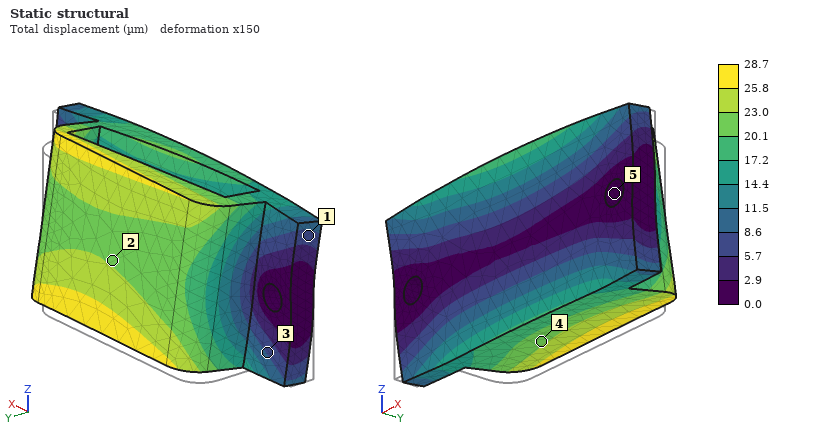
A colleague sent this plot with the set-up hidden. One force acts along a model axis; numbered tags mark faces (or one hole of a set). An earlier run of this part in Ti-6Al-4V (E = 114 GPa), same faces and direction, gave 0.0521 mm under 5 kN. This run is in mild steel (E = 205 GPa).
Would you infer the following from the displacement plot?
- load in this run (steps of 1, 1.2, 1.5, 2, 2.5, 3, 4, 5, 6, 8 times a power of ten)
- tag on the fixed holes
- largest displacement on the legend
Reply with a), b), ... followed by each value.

a) 5 kN
b) 5
c) 28.7 µm
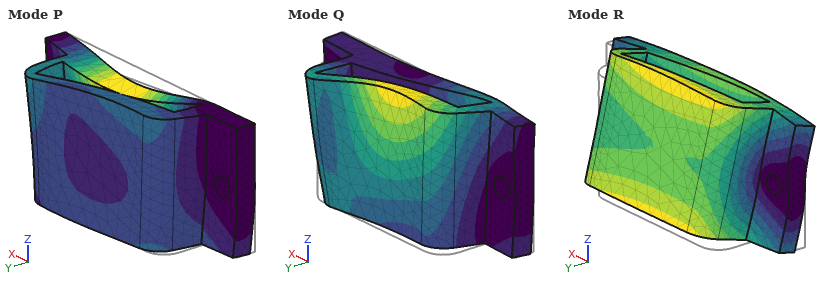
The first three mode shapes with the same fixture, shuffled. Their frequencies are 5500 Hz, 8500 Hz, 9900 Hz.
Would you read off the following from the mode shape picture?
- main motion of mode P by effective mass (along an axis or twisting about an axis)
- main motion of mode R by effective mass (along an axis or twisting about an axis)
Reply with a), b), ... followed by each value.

a) along Y
b) along Z
